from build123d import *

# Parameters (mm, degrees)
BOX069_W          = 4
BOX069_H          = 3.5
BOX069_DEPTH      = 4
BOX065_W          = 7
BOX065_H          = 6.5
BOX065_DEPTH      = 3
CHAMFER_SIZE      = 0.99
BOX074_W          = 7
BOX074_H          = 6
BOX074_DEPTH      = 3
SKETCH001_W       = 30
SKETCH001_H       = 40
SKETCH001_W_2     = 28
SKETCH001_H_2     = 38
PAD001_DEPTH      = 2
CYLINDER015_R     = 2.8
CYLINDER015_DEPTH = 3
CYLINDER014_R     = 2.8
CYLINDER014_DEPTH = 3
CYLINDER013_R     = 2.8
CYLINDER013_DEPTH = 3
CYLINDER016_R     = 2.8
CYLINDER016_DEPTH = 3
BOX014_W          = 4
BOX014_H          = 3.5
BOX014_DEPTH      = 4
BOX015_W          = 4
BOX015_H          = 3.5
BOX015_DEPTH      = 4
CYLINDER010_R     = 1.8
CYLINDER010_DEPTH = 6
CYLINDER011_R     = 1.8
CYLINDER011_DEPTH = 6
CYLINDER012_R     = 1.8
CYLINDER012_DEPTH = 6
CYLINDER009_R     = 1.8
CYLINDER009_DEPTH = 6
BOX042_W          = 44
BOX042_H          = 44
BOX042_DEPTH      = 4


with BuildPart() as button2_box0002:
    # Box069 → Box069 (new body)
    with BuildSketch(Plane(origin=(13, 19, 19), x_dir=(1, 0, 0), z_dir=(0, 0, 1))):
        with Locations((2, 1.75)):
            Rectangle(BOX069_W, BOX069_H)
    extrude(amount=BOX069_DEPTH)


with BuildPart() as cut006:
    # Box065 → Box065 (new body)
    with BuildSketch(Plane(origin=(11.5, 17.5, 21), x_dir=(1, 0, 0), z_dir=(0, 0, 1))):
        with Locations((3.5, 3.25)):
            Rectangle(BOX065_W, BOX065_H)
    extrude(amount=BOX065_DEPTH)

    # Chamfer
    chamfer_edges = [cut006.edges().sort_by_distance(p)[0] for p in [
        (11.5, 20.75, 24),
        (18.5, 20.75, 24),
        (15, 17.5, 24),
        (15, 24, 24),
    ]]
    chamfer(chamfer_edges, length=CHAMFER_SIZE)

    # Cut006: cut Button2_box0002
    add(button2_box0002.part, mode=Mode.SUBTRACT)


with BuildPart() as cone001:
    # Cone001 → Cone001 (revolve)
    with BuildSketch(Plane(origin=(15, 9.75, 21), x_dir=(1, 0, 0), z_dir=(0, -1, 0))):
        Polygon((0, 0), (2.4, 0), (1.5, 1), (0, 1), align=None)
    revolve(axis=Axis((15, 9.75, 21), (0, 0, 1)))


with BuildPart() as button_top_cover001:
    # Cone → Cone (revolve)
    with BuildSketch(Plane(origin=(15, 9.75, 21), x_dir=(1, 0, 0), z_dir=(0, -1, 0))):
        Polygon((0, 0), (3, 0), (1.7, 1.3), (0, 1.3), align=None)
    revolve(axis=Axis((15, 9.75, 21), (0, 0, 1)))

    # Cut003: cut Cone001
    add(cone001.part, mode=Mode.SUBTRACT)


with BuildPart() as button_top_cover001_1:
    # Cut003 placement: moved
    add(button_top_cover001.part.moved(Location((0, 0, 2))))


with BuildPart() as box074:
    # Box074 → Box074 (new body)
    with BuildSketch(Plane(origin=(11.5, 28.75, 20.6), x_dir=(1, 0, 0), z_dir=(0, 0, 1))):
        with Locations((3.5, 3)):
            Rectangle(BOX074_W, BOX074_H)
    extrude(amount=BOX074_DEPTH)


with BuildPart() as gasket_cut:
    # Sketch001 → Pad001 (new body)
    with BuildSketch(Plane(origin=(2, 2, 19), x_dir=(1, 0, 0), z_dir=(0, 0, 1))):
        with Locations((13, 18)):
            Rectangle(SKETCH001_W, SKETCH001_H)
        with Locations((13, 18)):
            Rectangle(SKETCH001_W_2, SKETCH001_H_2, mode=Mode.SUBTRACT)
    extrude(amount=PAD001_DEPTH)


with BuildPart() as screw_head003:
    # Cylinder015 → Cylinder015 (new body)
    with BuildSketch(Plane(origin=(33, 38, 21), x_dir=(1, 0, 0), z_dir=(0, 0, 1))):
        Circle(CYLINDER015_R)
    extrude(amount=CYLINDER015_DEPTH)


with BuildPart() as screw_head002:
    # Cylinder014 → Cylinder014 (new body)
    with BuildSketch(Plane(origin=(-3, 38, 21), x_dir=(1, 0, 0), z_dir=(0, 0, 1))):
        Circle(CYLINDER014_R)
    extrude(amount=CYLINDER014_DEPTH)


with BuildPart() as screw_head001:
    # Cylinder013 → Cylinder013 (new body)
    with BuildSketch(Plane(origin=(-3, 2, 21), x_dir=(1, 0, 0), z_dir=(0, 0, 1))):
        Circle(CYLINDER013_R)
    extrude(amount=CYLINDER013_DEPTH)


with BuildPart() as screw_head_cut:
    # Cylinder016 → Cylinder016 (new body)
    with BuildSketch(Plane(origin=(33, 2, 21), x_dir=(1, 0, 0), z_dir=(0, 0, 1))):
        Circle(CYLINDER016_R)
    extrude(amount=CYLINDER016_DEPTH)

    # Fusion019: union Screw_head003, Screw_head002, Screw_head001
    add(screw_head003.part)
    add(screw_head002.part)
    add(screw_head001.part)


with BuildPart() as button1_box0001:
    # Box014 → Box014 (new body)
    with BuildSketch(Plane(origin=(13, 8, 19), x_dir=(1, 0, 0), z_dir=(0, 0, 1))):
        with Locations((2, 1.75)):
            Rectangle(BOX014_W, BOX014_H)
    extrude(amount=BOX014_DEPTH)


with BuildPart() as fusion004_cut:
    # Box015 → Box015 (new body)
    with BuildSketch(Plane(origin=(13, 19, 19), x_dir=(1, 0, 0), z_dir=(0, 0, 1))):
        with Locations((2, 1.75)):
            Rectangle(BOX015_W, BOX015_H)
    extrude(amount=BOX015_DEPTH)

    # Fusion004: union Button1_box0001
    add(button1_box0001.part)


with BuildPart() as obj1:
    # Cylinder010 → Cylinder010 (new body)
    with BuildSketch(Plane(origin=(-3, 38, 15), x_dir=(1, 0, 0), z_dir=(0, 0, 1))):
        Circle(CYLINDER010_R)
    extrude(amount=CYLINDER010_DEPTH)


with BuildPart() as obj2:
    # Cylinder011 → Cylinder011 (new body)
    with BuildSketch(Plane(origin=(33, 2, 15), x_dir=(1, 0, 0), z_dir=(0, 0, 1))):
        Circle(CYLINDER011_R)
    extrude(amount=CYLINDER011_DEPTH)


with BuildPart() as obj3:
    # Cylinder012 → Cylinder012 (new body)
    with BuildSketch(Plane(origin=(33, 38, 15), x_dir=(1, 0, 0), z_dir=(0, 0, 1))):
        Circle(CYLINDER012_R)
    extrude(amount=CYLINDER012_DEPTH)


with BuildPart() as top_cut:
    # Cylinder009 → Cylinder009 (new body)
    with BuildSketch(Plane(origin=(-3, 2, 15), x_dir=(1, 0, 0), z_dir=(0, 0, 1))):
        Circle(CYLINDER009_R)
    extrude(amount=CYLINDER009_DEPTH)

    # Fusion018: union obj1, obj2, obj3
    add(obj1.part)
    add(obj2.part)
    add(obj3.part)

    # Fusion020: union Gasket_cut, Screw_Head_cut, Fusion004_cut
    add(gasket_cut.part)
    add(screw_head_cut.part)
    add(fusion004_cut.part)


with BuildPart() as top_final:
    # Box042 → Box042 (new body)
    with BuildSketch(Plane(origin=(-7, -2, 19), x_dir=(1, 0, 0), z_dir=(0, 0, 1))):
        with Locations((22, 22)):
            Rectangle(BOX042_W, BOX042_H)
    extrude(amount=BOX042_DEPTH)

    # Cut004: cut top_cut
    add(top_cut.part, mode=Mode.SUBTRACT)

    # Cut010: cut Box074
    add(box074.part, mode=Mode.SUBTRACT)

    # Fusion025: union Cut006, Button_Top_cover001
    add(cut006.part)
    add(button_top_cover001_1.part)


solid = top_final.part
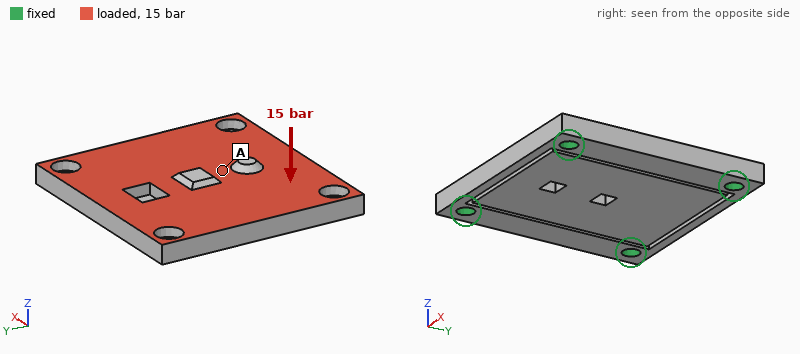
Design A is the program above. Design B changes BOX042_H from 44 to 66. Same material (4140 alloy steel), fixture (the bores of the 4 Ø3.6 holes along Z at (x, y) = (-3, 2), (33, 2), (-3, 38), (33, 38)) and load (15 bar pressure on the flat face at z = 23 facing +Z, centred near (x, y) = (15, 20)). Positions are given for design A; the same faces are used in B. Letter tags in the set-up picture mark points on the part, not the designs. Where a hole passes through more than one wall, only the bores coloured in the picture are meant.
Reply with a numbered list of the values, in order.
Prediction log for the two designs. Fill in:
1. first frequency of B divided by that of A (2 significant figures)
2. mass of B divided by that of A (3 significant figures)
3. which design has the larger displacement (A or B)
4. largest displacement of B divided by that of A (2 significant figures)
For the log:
1. 0.87
2. 1.55
3. B
4. 1.5
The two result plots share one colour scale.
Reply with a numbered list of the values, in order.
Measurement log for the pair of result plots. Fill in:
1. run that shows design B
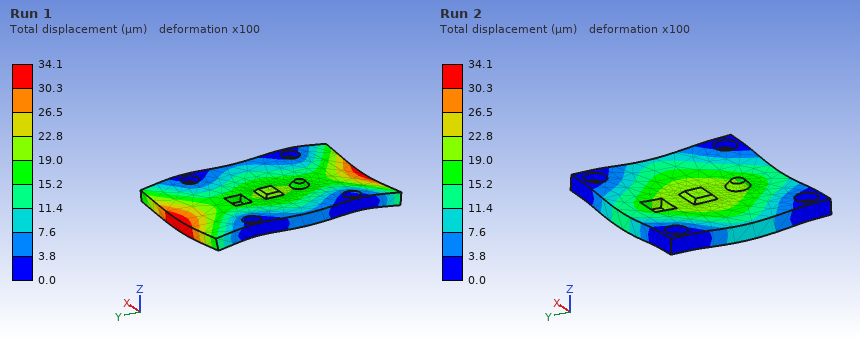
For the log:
1. Run 1
